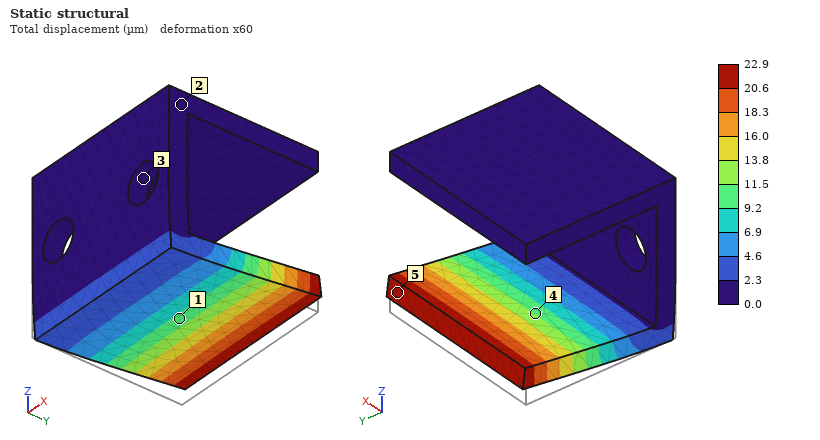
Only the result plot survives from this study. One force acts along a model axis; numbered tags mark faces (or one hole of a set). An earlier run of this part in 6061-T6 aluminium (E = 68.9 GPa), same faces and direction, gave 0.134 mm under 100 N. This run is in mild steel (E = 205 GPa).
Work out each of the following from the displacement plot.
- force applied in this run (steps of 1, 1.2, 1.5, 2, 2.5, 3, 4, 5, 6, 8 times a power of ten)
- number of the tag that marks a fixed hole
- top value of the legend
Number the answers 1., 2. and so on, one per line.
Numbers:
1. 50 N
2. 3
3. 22.9 µm
